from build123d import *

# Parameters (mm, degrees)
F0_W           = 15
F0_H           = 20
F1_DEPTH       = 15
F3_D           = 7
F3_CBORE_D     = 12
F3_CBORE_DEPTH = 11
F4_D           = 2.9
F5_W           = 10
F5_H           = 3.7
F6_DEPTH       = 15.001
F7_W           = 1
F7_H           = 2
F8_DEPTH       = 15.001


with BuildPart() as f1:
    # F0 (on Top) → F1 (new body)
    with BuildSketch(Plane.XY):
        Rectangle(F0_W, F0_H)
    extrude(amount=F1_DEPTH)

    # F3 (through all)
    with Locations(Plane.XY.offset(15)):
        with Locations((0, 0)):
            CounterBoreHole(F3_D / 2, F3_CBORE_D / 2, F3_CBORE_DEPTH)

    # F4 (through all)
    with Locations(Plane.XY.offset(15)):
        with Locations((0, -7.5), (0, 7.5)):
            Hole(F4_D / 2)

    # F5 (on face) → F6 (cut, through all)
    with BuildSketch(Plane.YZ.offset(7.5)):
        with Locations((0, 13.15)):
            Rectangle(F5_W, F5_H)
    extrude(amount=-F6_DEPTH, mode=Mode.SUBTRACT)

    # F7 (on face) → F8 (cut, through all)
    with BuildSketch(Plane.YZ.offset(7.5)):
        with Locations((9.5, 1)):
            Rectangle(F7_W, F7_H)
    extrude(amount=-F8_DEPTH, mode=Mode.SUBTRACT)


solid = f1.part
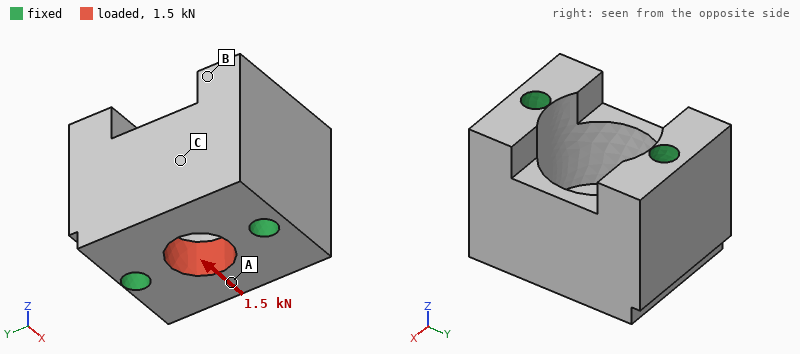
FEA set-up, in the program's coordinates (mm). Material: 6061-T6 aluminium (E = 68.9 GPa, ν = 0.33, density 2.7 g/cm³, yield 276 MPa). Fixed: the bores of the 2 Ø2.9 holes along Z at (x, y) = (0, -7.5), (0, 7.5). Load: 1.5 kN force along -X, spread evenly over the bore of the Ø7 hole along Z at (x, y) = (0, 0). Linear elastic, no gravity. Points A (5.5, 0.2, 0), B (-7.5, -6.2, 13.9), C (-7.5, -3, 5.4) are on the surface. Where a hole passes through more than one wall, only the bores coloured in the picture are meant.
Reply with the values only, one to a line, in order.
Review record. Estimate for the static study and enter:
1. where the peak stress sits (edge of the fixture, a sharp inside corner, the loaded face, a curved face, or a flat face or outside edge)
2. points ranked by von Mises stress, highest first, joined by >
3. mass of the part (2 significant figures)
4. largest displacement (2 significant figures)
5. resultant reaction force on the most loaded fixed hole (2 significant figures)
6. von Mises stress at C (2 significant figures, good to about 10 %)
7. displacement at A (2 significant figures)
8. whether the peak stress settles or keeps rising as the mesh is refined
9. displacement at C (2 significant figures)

edge of the fixture
A > C > B
7.3 g
4.2 µm
750 N
11 MPa
3.8 µm
keeps rising
1.5 µm
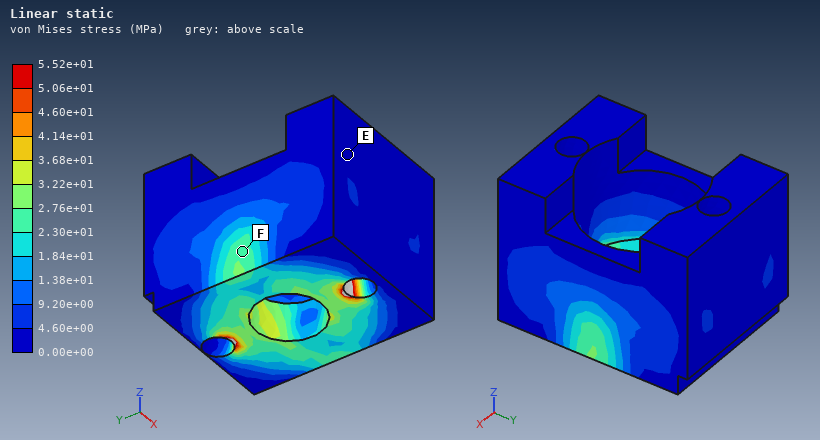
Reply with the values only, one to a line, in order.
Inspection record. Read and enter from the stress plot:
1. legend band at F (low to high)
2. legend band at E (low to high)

2.30e+01 to 2.76e+01 MPa
0.00e+00 to 4.60e+00 MPa
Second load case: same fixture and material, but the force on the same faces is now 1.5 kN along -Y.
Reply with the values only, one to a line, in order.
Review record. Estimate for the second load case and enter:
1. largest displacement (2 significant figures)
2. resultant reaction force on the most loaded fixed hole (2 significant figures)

2.4 µm
760 N
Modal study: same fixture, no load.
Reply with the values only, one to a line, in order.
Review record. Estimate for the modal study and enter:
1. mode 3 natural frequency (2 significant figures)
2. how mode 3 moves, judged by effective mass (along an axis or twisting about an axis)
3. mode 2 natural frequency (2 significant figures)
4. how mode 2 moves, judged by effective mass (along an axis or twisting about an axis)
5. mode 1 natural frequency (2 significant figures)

71 kHz
twisting about Y
62 kHz
along Y
59 kHz
